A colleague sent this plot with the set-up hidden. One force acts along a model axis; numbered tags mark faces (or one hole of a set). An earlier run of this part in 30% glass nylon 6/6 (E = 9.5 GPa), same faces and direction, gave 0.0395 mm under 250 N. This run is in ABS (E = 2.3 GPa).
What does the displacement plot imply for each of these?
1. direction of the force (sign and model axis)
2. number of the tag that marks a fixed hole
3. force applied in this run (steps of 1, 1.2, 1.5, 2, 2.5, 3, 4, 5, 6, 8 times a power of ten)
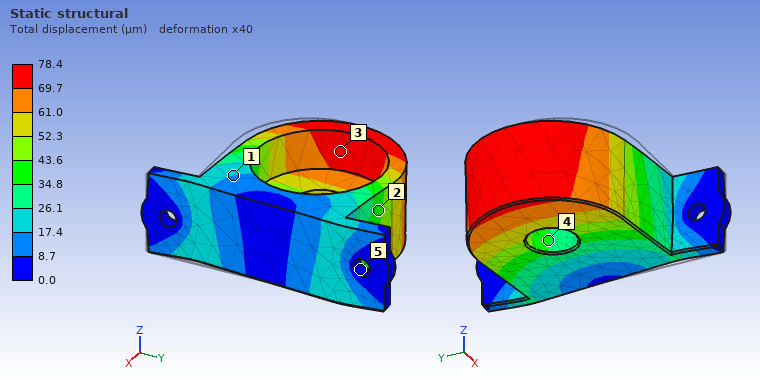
+Y
5
120 N
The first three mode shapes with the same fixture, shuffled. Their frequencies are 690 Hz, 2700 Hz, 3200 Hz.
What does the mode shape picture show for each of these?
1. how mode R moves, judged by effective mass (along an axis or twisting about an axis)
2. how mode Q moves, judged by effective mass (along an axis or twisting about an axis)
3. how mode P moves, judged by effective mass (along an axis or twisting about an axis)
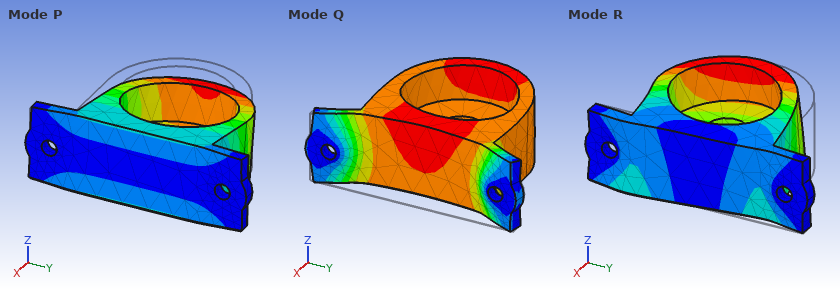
along Y
along X
along Z
